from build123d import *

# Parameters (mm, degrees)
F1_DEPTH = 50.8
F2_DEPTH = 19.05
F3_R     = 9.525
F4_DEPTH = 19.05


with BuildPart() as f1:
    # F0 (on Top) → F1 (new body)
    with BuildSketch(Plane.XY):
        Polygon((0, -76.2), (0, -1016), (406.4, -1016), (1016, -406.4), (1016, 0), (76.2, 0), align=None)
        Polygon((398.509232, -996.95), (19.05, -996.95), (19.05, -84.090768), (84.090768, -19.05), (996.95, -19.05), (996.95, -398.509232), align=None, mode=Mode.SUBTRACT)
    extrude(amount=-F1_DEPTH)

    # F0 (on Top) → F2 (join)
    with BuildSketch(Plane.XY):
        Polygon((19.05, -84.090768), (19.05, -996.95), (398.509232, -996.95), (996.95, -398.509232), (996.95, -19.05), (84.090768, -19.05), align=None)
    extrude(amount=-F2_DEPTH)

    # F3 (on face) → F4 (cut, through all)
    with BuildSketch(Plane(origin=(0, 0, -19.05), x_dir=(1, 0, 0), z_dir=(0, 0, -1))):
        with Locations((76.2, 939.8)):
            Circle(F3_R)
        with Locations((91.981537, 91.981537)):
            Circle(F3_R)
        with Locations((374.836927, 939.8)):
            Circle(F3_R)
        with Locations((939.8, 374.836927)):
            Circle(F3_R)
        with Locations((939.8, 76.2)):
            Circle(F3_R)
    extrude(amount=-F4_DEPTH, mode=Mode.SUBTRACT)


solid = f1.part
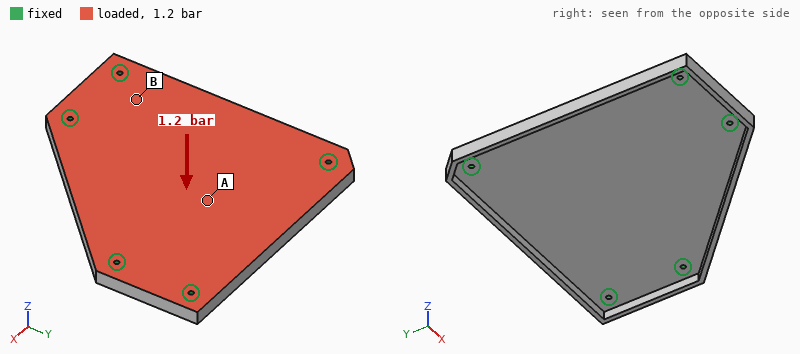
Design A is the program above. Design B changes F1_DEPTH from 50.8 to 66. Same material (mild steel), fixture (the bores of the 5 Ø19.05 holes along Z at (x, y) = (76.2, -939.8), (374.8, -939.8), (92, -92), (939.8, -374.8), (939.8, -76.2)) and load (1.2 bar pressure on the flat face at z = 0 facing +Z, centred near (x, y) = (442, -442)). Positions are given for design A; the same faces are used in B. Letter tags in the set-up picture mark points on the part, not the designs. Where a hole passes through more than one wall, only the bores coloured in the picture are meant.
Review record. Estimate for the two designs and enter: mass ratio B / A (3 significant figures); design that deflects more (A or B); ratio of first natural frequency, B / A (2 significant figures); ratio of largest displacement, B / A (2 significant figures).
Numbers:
1.06
A
1.1
0.90
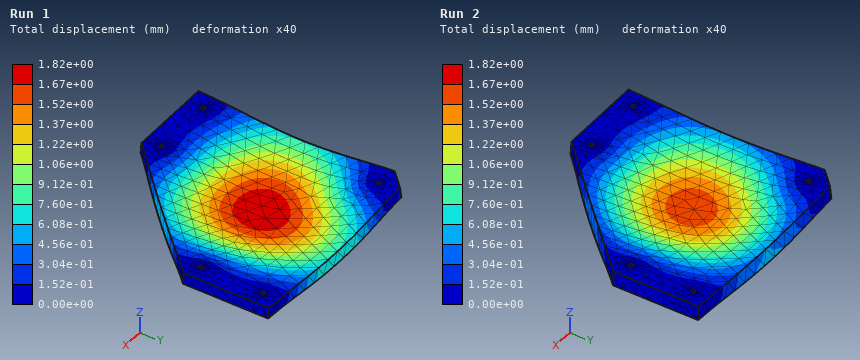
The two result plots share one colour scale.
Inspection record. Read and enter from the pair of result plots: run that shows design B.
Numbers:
Run 2
